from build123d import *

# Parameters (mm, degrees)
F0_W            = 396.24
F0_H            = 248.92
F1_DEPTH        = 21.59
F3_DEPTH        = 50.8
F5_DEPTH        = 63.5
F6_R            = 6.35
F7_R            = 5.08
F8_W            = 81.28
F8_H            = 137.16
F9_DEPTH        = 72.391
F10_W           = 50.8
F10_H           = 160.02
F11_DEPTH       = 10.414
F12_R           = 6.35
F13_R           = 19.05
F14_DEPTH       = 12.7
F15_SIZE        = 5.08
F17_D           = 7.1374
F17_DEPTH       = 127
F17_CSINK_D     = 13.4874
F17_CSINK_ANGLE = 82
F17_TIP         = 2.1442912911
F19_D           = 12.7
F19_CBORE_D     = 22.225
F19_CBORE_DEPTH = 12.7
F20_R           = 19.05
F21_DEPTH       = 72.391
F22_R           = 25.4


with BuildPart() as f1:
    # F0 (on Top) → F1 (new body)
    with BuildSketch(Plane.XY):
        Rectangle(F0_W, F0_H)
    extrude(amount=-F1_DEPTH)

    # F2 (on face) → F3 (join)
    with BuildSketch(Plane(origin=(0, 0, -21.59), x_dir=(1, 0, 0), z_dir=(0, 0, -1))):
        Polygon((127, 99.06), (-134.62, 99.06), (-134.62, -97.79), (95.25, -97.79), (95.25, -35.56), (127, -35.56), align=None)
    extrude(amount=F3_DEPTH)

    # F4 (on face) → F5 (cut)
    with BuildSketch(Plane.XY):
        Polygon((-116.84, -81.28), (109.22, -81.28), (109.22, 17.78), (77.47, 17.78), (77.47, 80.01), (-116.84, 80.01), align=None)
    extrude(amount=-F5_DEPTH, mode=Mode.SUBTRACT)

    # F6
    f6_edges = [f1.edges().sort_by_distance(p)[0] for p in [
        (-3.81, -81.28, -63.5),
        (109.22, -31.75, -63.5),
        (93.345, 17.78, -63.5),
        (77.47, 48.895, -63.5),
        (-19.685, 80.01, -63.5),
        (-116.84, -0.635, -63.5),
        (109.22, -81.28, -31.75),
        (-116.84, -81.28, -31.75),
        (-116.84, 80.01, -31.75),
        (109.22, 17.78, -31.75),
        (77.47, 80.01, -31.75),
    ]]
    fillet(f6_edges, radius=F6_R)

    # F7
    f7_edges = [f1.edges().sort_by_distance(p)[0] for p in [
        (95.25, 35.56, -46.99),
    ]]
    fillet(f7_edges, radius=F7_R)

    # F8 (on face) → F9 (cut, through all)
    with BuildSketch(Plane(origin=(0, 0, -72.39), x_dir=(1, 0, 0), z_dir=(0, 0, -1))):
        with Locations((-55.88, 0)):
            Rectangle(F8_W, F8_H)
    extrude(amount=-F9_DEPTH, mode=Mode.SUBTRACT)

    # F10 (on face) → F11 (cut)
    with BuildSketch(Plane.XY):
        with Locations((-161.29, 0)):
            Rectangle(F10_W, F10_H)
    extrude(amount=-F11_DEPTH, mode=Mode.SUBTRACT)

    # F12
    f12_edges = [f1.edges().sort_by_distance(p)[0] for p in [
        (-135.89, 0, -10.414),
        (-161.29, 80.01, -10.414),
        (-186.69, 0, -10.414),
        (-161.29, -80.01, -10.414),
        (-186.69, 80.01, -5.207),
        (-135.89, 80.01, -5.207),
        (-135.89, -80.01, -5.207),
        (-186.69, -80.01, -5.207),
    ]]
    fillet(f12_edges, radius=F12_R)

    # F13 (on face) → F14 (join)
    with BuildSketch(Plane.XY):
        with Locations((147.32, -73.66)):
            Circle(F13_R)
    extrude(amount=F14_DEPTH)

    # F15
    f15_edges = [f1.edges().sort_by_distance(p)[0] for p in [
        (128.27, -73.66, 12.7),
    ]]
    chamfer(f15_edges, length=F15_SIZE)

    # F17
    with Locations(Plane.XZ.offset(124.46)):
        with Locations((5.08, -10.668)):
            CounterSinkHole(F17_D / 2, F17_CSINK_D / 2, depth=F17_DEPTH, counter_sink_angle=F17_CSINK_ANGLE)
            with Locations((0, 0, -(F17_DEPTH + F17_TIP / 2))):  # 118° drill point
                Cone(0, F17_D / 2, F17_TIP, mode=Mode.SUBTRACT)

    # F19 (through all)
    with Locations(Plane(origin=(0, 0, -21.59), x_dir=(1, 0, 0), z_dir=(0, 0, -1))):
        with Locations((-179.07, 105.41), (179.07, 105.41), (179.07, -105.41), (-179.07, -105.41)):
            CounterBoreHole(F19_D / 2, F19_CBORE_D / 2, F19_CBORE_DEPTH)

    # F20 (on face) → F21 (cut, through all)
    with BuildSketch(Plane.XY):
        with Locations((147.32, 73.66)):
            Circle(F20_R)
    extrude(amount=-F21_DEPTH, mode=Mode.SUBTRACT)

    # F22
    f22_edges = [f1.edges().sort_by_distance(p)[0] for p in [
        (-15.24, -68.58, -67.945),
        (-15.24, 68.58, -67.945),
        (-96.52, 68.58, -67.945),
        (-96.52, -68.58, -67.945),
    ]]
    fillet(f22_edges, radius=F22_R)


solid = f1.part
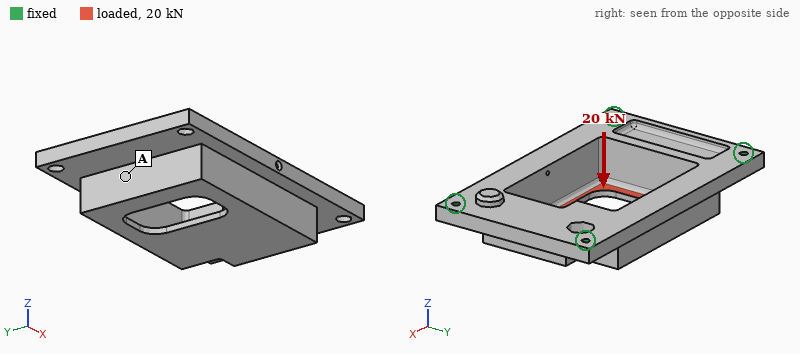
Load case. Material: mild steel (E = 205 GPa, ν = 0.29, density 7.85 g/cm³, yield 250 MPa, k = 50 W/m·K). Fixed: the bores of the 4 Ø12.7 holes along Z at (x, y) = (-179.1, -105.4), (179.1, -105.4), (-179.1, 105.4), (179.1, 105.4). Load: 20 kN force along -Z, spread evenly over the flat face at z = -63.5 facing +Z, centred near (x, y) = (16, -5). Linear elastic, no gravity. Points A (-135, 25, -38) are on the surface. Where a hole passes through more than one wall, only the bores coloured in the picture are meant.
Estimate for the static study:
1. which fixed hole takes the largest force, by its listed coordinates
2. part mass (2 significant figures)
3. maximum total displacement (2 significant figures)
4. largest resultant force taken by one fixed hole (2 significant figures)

(179.1, -105.4)
18 kg
0.18 mm
11 kN
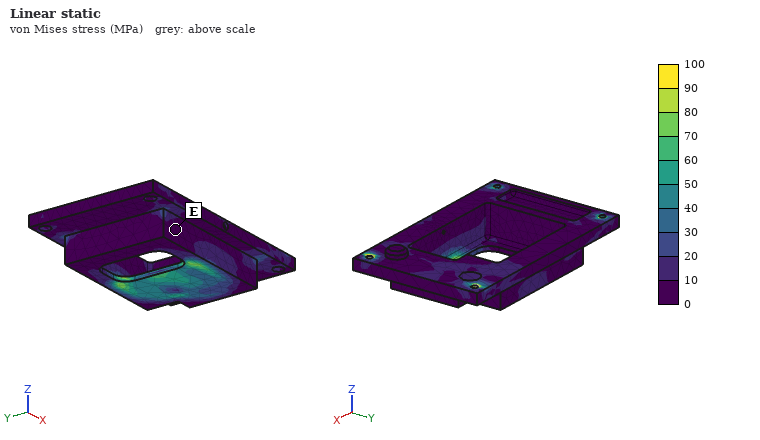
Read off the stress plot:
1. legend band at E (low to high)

0 to 10 MPa
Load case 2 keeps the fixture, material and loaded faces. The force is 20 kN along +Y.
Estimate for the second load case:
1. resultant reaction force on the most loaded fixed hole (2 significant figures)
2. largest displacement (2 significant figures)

9.8 kN
36 µm
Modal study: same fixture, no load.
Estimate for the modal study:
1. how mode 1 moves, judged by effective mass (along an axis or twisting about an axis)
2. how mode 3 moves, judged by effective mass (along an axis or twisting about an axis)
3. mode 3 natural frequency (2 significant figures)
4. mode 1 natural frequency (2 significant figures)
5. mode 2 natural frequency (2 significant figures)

along Z
twisting about Y
1700 Hz
980 Hz
1300 Hz
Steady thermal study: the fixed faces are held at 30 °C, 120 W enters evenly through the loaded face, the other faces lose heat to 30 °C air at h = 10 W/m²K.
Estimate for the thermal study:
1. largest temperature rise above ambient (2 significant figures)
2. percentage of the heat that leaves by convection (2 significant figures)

63 K
50 %
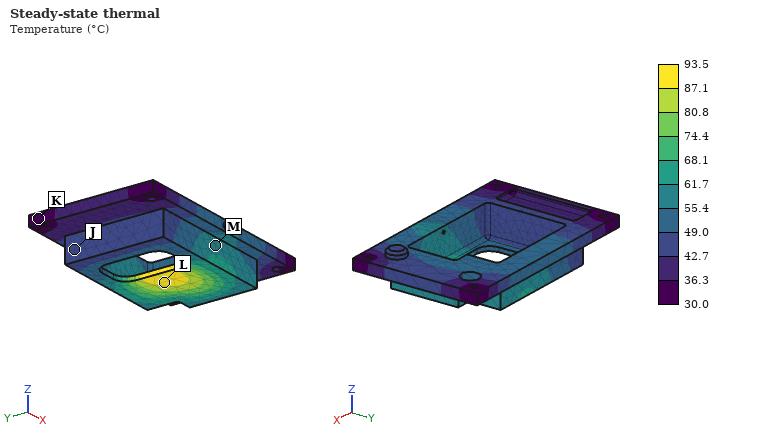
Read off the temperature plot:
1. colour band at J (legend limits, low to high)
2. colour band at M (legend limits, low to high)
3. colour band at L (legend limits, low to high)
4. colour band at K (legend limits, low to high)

42.7 to 49.0 °C
55.4 to 61.7 °C
87.1 to 93.5 °C
30.0 to 36.3 °C
